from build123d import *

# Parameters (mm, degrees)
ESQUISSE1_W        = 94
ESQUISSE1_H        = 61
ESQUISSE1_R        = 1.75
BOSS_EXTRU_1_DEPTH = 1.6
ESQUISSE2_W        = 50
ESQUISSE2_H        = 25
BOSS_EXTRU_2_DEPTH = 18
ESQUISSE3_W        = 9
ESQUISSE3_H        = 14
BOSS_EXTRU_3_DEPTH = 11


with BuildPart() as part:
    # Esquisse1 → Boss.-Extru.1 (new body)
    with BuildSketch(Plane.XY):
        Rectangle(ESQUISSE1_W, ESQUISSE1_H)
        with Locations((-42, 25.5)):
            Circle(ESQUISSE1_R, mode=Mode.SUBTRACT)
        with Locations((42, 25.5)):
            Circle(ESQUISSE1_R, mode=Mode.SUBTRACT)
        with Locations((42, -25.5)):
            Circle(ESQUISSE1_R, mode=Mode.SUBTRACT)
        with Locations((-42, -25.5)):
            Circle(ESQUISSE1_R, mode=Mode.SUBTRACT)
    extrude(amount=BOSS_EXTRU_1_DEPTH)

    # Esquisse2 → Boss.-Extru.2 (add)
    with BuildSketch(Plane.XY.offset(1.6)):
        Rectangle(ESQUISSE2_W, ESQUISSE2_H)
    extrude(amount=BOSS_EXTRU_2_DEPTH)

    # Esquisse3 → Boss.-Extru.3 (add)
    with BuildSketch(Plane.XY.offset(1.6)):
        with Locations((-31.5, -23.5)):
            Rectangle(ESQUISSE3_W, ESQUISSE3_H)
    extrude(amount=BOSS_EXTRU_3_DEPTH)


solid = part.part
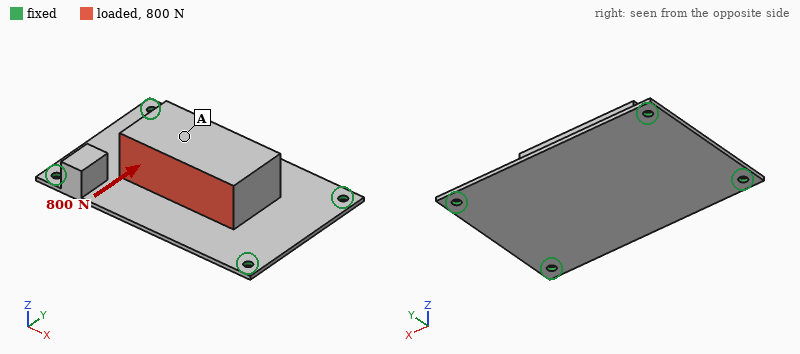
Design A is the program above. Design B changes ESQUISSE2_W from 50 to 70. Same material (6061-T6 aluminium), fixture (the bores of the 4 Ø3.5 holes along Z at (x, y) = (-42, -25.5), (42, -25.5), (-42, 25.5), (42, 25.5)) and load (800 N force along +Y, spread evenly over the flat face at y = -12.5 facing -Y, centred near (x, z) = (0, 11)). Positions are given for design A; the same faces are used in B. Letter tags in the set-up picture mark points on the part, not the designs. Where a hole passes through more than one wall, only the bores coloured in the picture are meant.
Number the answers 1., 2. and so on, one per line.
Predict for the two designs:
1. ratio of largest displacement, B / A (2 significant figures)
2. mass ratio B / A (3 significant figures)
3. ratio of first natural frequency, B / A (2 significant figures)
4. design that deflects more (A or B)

1. 0.43
2. 1.27
3. 1.3
4. A
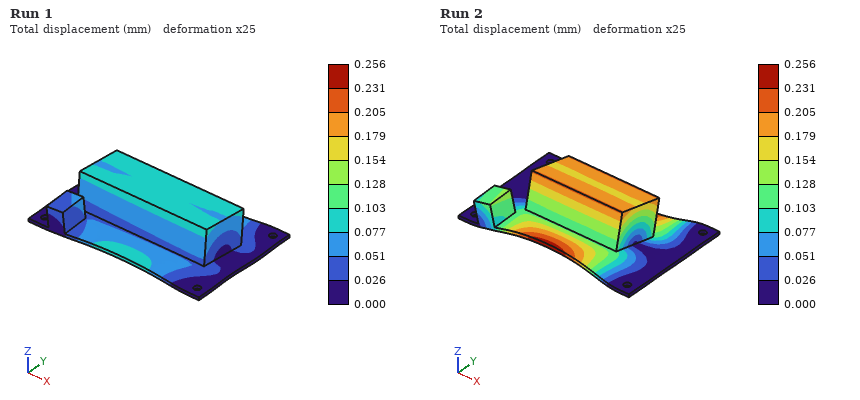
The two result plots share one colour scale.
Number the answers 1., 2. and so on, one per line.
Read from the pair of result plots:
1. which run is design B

1. Run 1
